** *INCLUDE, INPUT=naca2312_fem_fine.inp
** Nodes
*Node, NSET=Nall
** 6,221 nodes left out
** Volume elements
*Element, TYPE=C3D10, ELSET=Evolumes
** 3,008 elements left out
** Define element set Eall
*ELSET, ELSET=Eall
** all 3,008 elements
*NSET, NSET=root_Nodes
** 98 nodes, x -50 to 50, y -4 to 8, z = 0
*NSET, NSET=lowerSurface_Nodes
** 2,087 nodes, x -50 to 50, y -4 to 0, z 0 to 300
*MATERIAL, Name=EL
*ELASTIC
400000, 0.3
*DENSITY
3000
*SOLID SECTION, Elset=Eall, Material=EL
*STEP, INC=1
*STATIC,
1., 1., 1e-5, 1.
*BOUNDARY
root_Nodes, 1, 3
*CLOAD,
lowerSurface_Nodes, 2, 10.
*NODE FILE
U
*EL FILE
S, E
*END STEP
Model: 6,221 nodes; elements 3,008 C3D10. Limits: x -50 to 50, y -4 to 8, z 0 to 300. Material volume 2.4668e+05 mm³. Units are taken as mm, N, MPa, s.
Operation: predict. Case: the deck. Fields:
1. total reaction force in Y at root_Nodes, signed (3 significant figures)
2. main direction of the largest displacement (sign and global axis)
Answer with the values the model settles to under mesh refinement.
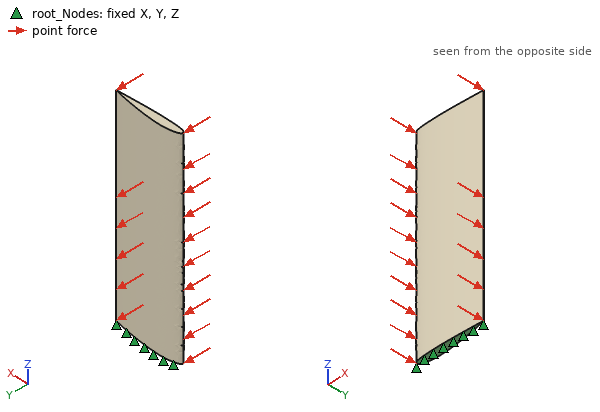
-20900 N
+Y
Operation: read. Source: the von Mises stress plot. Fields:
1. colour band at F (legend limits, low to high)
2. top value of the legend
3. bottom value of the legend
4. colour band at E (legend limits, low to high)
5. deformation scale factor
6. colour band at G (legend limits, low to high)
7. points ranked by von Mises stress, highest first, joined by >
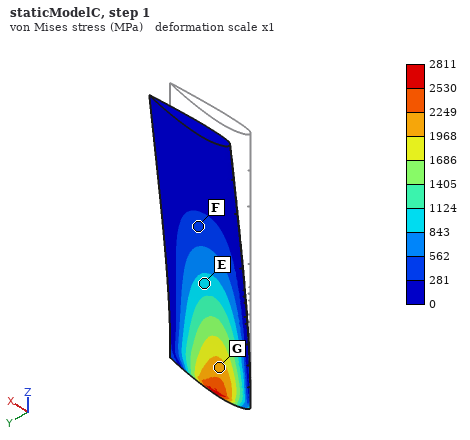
281 to 562 MPa
2811 MPa
0 MPa
843 to 1124 MPa
1
1968 to 2249 MPa
G > E > F
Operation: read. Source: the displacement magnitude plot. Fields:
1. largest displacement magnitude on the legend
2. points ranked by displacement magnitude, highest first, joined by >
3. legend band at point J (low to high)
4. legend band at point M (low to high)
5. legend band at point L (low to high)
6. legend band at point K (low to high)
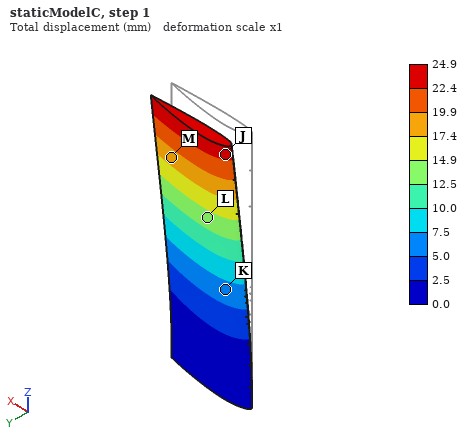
24.9 mm
J > M > L > K
22.4 to 24.9 mm
17.4 to 19.9 mm
12.5 to 14.9 mm
5.0 to 7.5 mm
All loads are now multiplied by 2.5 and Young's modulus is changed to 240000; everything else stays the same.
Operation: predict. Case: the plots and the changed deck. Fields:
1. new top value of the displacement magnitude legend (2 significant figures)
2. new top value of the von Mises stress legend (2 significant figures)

100 mm
7000 MPa
